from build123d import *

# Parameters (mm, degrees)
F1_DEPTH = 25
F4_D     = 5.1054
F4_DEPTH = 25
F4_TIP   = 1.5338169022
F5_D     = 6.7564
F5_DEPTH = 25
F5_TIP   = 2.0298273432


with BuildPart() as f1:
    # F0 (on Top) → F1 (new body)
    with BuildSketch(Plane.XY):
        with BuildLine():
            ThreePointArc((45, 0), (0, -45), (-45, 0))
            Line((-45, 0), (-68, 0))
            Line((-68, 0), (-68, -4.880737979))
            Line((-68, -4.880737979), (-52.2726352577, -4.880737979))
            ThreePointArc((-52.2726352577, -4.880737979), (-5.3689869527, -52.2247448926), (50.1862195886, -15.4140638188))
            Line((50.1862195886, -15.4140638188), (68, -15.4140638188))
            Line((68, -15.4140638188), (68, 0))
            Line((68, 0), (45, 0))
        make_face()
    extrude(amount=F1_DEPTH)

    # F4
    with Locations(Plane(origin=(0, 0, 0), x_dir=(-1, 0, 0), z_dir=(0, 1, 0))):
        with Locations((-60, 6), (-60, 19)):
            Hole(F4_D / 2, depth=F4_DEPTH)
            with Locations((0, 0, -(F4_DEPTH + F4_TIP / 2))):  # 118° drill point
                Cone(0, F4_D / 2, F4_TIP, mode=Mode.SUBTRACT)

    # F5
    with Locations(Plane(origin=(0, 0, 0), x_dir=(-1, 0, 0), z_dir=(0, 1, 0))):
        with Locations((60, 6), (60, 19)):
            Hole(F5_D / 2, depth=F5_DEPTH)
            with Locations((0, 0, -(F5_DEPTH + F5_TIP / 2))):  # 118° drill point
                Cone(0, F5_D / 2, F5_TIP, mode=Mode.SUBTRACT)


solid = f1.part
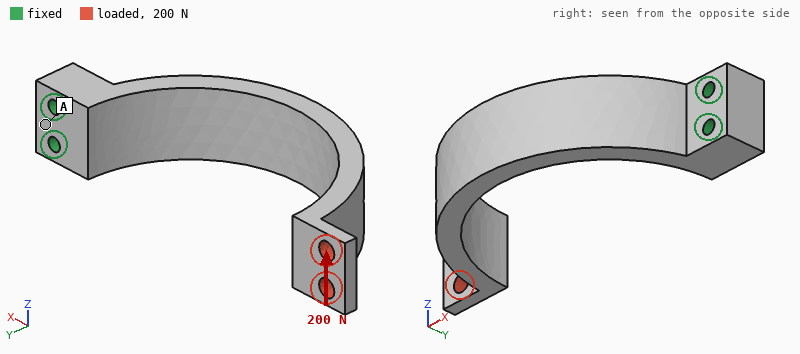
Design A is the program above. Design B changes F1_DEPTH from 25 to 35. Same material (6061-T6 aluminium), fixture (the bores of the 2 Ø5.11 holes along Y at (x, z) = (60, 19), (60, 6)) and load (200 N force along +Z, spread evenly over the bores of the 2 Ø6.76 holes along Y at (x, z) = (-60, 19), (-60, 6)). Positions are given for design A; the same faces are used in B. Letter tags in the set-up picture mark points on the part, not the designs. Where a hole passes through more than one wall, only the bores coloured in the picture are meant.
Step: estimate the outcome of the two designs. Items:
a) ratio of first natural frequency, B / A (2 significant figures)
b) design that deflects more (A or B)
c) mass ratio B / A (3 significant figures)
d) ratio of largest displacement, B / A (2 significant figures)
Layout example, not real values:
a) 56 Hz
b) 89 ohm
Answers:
a) 1.00
b) A
c) 1.41
d) 0.63
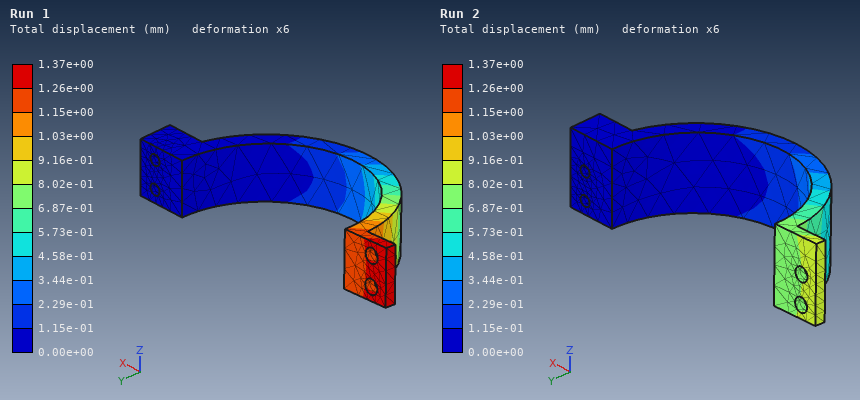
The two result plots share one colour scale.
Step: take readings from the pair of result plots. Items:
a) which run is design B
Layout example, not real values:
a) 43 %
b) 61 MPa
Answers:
a) Run 2
